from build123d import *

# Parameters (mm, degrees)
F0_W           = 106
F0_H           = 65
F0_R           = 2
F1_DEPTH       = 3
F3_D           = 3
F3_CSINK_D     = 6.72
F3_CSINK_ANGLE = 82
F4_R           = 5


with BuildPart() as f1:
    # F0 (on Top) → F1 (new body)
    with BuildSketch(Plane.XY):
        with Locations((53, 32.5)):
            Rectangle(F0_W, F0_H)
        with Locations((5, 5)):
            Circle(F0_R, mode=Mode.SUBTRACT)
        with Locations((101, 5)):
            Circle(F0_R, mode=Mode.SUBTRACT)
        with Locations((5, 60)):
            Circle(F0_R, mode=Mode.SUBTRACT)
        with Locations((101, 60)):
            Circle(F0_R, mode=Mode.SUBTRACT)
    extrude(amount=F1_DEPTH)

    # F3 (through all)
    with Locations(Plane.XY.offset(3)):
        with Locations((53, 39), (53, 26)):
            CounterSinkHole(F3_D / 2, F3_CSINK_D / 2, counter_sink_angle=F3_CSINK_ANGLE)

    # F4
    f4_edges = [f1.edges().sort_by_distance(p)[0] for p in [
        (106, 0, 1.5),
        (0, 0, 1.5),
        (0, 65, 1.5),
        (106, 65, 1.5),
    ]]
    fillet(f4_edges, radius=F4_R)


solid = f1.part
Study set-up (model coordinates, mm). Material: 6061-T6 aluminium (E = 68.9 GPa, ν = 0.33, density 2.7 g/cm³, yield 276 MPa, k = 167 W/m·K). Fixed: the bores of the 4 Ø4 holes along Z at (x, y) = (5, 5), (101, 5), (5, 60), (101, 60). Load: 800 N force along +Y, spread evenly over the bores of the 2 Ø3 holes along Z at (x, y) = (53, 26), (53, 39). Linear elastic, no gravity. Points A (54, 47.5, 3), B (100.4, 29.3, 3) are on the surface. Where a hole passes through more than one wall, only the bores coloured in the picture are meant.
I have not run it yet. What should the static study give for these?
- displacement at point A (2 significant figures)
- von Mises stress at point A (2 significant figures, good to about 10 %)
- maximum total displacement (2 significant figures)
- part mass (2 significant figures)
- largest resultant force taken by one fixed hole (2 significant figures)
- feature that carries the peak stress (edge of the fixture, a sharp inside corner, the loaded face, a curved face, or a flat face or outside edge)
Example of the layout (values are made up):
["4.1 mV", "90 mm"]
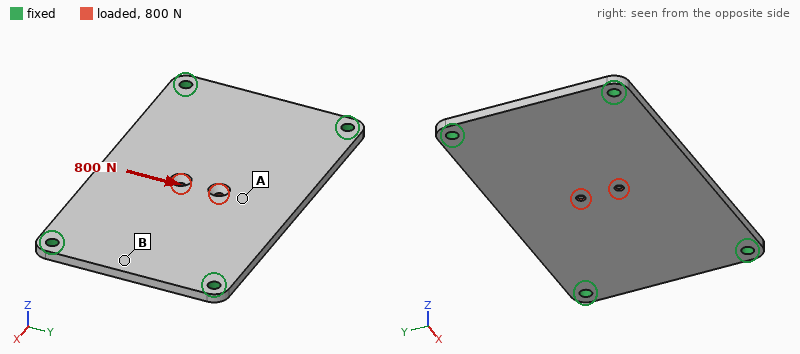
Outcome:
["11 µm", "6.5 MPa", "17 µm", "55 g", "260 N", "the loaded face"]
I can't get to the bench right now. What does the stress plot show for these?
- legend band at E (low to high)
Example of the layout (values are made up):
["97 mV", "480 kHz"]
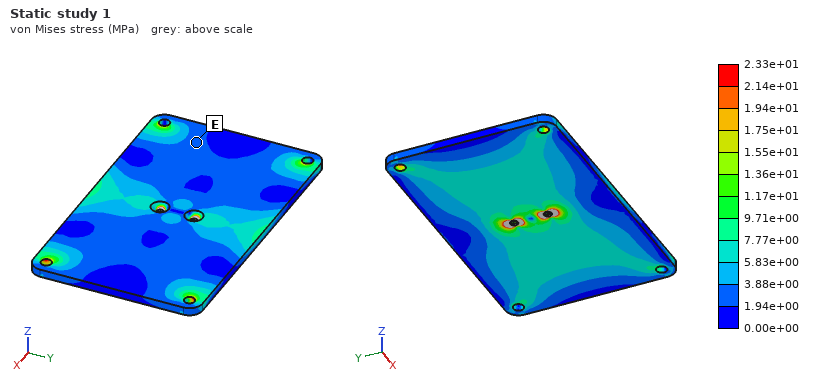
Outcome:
["1.94e+00 to 3.88e+00 MPa"]
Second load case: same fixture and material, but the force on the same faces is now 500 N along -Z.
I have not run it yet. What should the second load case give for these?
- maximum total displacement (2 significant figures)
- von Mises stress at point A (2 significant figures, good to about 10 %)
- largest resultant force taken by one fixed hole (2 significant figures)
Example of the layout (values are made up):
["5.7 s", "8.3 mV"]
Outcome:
["0.34 mm", "69 MPa", "130 N"]
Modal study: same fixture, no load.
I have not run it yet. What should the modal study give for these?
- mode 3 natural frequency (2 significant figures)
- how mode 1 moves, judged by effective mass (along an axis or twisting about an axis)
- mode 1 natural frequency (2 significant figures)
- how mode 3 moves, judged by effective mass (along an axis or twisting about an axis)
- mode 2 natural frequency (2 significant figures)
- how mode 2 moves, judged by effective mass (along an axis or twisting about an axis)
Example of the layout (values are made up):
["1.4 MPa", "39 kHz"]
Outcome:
["3800 Hz", "along Z", "1400 Hz", "twisting about Y", "2400 Hz", "twisting about X"]
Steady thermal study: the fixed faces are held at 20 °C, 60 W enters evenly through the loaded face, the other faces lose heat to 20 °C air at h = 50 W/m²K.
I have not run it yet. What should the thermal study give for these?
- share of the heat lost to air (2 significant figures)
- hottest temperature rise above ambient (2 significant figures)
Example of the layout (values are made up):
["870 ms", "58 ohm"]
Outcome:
["28 %", "76 K"]
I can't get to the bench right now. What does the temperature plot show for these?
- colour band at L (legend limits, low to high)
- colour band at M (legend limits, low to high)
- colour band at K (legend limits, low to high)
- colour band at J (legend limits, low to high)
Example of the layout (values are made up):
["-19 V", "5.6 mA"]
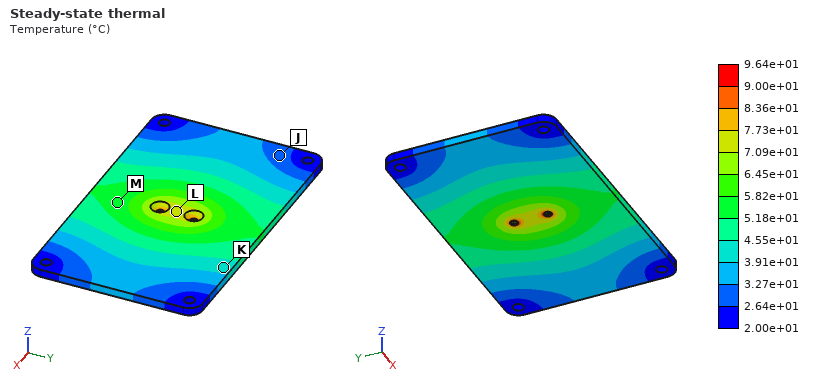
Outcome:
["7.09e+01 to 7.73e+01 °C", "5.18e+01 to 5.82e+01 °C", "3.91e+01 to 4.55e+01 °C", "2.64e+01 to 3.27e+01 °C"]
